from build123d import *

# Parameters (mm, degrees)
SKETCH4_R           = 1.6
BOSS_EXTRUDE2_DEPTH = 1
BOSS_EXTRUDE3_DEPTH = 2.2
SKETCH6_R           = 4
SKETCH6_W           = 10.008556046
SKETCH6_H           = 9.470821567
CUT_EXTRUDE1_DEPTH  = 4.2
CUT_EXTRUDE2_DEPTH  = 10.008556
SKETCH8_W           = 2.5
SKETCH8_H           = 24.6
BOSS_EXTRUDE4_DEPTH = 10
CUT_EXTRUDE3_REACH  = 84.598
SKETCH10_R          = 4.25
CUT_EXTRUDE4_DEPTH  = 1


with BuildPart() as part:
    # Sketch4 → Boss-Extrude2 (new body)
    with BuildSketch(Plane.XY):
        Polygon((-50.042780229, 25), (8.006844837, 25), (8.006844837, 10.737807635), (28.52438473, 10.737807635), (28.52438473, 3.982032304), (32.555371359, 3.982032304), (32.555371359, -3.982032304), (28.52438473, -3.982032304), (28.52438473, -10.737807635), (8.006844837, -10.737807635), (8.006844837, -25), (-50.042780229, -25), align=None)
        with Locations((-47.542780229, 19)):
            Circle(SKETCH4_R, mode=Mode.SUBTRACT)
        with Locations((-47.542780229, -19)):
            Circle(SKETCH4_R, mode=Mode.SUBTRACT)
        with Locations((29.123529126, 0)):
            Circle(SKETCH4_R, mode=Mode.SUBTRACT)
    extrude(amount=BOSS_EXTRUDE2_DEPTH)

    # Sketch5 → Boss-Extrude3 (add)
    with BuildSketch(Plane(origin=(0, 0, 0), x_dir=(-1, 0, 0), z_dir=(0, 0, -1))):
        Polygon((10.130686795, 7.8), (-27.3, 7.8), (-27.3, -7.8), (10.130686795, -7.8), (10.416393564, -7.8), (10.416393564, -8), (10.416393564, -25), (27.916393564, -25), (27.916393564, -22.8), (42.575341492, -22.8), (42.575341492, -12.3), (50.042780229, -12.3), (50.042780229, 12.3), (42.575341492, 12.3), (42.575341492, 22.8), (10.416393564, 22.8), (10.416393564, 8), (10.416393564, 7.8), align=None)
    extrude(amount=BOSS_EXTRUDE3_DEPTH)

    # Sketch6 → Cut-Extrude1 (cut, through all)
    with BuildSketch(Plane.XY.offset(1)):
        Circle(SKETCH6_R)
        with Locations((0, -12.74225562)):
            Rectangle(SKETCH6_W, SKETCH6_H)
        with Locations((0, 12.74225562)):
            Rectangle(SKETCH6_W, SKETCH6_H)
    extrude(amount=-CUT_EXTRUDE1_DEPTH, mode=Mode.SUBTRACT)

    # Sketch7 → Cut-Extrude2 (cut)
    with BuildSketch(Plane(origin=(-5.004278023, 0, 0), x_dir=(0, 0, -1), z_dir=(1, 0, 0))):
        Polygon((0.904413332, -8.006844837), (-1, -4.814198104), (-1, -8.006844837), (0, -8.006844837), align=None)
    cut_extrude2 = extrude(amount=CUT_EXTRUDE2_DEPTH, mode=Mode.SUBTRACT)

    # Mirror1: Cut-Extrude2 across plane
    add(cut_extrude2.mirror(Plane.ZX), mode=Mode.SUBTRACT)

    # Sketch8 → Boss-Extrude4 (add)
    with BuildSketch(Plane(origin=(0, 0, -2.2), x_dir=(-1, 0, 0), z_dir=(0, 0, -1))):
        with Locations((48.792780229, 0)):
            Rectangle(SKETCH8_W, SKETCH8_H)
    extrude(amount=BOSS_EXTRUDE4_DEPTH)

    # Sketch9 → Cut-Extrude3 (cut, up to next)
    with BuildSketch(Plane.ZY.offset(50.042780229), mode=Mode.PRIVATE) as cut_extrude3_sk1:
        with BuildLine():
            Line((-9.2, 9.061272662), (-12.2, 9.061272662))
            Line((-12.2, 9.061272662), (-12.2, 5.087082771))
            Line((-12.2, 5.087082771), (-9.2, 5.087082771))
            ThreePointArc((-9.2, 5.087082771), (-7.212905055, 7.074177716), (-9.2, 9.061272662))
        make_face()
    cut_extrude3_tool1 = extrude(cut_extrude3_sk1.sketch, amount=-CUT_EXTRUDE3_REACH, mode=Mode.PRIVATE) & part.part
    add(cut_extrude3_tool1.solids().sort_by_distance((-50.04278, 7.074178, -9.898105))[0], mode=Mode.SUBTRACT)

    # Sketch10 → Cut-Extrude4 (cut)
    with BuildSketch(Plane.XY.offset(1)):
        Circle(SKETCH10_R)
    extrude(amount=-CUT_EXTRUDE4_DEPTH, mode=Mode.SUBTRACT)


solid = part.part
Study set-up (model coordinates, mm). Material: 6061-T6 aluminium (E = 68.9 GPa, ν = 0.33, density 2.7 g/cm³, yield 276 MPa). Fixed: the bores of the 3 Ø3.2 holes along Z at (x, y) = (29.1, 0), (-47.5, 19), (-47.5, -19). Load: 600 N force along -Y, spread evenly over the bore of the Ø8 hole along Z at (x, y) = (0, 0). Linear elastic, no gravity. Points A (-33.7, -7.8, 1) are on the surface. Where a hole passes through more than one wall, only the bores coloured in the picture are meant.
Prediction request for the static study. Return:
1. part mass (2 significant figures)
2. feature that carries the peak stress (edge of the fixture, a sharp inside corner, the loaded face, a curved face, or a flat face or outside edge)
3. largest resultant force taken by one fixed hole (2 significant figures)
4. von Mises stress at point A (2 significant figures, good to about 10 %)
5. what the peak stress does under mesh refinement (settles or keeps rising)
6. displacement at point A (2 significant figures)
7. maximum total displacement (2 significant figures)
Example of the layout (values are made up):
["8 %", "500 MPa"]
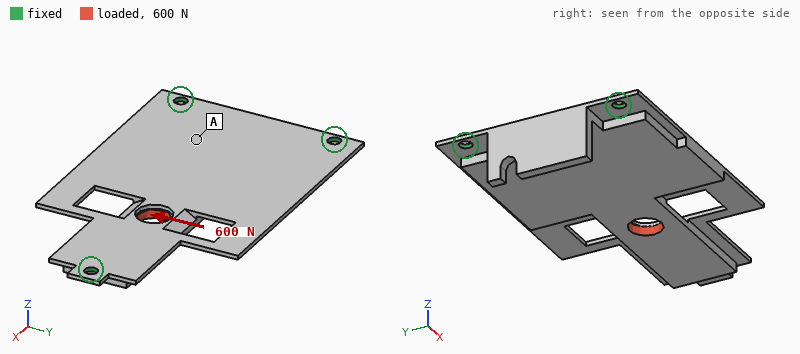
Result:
["23 g", "edge of the fixture", "430 N", "8.7 MPa", "keeps rising", "7.2 µm", "28 µm"]
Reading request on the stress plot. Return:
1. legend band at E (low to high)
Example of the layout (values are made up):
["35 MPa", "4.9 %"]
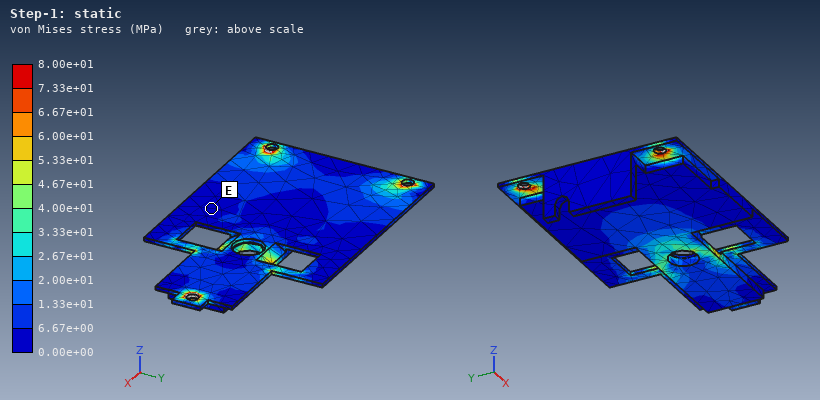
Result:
["0.00e+00 to 6.67e+00 MPa"]
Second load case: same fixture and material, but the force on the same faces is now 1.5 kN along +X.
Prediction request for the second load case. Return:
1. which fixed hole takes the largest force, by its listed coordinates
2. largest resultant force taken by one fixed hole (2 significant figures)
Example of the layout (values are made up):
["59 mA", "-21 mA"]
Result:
["(29.1, 0)", "690 N"]
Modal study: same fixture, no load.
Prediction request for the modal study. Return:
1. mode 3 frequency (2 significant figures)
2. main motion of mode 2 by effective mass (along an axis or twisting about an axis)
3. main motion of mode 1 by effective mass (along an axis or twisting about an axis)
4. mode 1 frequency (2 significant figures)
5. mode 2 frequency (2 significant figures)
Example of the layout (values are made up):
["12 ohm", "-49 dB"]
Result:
["4200 Hz", "twisting about X", "along Z", "1400 Hz", "2500 Hz"]
